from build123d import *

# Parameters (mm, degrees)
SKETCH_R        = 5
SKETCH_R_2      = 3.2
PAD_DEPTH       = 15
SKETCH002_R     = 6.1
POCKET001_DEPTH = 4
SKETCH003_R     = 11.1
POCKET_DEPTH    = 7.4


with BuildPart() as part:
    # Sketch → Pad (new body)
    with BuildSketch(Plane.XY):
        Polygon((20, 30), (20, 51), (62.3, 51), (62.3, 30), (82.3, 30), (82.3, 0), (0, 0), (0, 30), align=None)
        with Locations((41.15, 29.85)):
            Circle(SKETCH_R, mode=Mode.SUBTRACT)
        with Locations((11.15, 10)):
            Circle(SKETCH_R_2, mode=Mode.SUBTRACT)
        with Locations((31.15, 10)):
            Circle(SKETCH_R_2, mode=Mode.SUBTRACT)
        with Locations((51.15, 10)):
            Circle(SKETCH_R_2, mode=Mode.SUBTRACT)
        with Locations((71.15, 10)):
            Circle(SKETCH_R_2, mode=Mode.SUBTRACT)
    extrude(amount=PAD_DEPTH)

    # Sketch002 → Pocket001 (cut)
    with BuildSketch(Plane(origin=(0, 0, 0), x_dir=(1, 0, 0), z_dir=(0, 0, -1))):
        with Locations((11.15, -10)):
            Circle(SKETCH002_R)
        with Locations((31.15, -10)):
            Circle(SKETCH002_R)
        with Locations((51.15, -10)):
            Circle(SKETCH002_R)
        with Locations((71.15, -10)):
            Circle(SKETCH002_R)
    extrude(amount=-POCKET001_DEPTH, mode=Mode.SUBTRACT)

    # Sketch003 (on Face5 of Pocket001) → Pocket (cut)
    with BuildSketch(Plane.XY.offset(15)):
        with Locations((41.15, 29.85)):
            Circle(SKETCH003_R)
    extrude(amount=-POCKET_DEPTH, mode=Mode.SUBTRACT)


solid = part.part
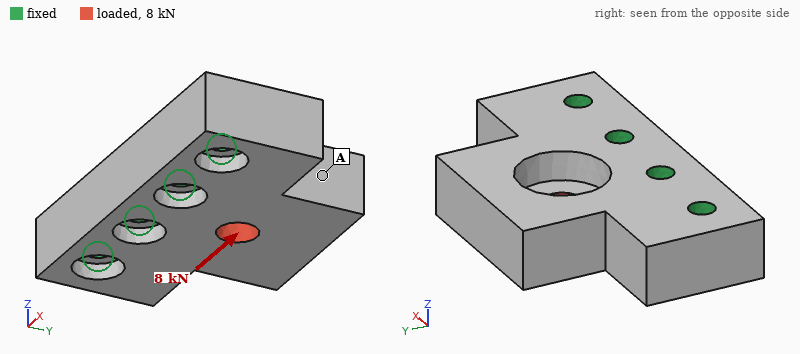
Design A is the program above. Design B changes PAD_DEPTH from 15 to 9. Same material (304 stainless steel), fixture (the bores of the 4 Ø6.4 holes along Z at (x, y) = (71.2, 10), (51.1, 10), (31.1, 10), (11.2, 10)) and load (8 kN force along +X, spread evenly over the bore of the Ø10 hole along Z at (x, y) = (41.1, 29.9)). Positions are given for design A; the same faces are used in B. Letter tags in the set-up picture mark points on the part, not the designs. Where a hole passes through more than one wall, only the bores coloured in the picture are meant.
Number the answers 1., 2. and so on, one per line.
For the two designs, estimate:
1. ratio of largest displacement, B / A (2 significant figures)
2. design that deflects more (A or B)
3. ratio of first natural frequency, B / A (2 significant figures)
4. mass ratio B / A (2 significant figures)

1. 1.3
2. B
3. 0.62
4. 0.61
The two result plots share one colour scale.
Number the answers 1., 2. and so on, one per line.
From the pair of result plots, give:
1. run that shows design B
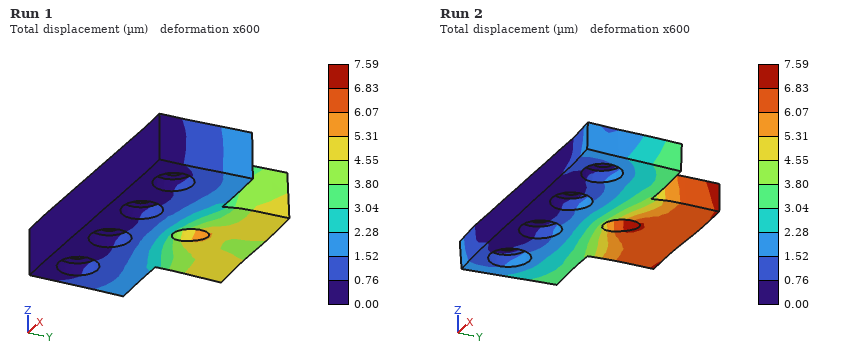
1. Run 2
